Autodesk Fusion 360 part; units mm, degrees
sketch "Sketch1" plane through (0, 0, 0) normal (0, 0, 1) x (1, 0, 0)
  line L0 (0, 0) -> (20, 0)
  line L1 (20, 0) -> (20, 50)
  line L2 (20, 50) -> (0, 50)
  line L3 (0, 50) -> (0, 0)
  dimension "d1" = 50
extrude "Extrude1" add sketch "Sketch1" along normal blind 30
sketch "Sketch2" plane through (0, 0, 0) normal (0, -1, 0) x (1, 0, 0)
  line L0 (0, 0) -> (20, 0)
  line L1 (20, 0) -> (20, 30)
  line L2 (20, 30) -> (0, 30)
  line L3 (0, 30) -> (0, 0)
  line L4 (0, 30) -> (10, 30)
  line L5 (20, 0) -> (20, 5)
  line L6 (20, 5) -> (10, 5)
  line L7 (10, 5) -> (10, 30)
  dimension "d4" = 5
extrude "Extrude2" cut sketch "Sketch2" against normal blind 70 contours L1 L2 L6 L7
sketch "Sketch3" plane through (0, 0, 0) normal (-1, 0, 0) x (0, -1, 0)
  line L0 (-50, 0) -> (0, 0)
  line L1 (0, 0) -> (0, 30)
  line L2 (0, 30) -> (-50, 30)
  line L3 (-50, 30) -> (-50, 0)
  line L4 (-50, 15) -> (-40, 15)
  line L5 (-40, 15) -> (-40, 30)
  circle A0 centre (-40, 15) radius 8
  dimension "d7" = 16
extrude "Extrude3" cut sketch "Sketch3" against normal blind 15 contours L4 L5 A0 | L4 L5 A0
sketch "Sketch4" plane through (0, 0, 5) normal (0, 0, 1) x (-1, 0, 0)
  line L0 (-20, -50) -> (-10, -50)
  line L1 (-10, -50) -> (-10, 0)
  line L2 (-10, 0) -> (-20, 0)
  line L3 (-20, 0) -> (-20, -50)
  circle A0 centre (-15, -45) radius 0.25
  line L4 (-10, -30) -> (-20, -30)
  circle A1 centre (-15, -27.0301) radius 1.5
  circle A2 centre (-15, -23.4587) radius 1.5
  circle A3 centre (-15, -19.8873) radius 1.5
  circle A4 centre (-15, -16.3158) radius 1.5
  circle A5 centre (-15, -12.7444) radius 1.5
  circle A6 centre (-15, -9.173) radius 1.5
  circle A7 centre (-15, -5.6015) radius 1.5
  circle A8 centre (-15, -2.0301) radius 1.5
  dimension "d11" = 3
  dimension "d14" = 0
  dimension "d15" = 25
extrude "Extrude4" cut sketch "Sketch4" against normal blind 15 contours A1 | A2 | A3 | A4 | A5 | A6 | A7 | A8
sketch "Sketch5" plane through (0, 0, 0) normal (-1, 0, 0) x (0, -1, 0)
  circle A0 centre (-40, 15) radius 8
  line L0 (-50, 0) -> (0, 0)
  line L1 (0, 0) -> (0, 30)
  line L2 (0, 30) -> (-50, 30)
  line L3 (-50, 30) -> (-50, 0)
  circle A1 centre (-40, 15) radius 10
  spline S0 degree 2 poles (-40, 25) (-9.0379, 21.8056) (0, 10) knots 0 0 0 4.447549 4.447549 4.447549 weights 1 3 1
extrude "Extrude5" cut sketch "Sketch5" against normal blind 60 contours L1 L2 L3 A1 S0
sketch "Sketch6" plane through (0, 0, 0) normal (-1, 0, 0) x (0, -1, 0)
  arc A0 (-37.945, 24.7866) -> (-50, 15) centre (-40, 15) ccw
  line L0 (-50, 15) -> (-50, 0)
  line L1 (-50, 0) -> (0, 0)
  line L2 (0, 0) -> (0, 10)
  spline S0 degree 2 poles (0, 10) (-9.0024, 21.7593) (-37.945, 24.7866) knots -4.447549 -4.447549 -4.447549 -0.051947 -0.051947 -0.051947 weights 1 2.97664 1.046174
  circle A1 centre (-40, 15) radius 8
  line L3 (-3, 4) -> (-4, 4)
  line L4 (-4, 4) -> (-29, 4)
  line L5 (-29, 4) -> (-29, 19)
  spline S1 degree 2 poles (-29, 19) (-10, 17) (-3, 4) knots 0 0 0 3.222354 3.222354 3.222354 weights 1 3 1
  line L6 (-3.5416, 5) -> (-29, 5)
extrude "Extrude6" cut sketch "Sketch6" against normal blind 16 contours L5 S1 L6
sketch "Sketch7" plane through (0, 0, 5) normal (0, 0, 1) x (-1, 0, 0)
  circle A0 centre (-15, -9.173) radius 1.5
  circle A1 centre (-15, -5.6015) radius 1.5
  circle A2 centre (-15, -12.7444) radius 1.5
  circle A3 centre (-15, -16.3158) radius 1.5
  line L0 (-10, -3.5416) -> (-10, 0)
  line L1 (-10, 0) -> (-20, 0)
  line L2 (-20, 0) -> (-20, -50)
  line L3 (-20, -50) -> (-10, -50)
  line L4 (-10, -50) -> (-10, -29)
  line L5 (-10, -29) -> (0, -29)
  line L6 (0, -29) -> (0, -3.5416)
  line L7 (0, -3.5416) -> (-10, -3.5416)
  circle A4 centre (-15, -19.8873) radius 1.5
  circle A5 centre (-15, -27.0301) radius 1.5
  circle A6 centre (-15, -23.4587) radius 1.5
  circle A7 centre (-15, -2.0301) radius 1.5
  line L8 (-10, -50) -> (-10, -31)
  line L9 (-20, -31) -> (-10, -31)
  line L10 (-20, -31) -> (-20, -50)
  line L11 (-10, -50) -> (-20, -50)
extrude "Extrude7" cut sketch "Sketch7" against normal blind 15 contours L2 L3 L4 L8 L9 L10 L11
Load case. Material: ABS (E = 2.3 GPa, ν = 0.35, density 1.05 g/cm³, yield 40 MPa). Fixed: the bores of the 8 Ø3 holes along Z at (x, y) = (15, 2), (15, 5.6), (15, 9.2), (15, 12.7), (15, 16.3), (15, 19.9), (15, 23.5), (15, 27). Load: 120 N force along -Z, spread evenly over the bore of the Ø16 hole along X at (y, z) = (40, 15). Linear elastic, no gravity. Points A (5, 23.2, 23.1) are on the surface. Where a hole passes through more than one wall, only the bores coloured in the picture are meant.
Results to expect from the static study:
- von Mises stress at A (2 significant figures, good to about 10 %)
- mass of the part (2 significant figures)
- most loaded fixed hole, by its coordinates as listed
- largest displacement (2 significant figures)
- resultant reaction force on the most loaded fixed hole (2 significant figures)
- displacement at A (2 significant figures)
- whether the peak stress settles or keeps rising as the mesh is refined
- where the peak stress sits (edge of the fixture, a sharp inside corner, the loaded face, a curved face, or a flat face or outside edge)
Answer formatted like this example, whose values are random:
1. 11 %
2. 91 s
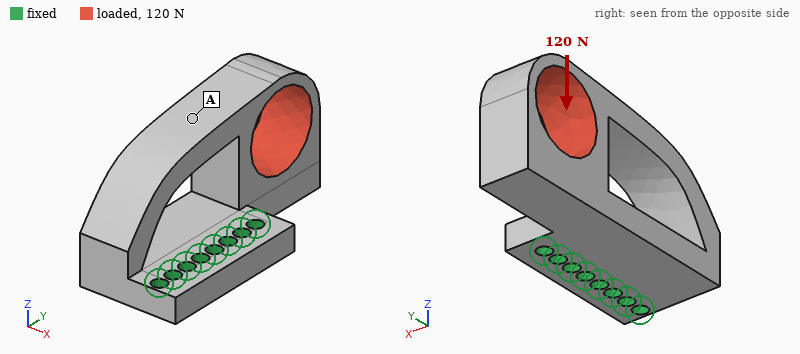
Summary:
1. 3.4 MPa
2. 7.7 g
3. (15, 27)
4. 0.66 mm
5. 130 N
6. 0.31 mm
7. keeps rising
8. edge of the fixture
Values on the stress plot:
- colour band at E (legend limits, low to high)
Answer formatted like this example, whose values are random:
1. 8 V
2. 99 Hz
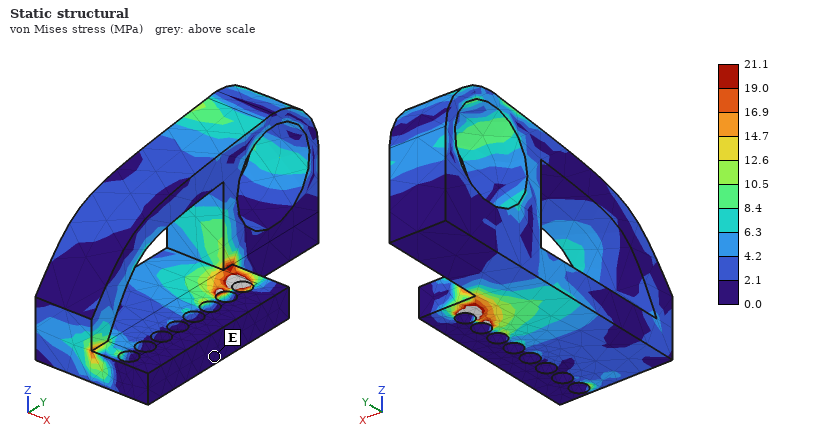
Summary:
1. 0.0 to 2.1 MPa
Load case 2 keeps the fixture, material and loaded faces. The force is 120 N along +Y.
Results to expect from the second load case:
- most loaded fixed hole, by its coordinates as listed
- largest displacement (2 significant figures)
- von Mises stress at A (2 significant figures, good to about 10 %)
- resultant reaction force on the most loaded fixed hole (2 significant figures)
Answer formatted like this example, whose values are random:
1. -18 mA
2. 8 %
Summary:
1. (15, 27)
2. 0.31 mm
3. 3.1 MPa
4. 67 N
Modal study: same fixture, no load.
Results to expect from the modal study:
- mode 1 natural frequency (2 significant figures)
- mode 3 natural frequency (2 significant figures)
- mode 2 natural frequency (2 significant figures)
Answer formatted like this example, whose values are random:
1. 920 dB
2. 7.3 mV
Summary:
1. 1200 Hz
2. 2500 Hz
3. 1600 Hz
